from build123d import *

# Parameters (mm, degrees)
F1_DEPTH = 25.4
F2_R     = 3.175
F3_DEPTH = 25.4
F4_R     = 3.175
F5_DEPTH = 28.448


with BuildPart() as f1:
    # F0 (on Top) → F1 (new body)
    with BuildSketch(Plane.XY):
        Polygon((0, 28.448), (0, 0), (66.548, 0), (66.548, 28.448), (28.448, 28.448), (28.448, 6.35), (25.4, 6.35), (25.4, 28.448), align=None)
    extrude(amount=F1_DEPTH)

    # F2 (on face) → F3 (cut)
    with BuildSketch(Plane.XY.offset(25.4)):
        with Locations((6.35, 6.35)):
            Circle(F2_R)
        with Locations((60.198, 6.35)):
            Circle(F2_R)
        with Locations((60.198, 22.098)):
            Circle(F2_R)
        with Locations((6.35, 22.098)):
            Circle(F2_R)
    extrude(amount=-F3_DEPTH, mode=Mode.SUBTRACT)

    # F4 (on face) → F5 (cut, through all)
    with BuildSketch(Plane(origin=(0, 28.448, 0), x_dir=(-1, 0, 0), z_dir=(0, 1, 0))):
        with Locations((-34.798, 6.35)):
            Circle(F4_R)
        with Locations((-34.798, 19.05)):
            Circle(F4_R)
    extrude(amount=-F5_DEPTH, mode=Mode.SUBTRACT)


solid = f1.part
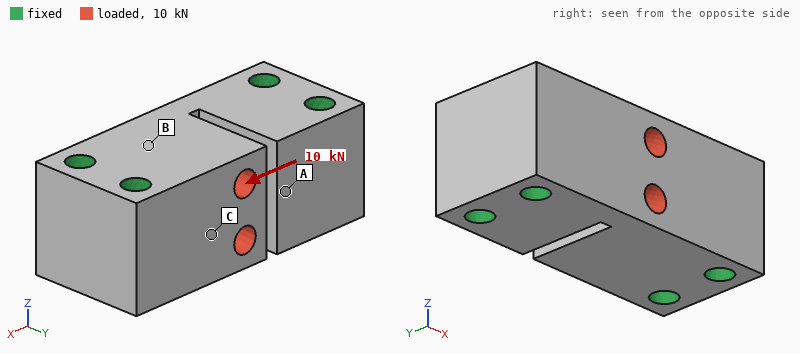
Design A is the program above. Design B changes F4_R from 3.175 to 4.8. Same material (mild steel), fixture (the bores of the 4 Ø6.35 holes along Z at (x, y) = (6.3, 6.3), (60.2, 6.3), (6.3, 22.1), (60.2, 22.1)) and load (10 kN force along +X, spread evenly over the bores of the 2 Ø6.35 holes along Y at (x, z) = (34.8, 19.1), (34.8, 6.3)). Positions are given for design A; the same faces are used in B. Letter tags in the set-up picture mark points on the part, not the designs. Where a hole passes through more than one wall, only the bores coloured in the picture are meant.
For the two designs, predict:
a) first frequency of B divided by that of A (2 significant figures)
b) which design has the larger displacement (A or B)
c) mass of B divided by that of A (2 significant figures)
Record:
1.0
B
0.94
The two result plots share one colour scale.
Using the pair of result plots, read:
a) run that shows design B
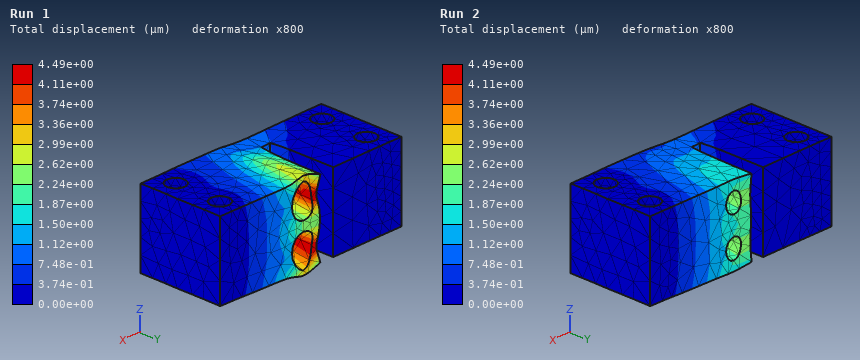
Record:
Run 1
